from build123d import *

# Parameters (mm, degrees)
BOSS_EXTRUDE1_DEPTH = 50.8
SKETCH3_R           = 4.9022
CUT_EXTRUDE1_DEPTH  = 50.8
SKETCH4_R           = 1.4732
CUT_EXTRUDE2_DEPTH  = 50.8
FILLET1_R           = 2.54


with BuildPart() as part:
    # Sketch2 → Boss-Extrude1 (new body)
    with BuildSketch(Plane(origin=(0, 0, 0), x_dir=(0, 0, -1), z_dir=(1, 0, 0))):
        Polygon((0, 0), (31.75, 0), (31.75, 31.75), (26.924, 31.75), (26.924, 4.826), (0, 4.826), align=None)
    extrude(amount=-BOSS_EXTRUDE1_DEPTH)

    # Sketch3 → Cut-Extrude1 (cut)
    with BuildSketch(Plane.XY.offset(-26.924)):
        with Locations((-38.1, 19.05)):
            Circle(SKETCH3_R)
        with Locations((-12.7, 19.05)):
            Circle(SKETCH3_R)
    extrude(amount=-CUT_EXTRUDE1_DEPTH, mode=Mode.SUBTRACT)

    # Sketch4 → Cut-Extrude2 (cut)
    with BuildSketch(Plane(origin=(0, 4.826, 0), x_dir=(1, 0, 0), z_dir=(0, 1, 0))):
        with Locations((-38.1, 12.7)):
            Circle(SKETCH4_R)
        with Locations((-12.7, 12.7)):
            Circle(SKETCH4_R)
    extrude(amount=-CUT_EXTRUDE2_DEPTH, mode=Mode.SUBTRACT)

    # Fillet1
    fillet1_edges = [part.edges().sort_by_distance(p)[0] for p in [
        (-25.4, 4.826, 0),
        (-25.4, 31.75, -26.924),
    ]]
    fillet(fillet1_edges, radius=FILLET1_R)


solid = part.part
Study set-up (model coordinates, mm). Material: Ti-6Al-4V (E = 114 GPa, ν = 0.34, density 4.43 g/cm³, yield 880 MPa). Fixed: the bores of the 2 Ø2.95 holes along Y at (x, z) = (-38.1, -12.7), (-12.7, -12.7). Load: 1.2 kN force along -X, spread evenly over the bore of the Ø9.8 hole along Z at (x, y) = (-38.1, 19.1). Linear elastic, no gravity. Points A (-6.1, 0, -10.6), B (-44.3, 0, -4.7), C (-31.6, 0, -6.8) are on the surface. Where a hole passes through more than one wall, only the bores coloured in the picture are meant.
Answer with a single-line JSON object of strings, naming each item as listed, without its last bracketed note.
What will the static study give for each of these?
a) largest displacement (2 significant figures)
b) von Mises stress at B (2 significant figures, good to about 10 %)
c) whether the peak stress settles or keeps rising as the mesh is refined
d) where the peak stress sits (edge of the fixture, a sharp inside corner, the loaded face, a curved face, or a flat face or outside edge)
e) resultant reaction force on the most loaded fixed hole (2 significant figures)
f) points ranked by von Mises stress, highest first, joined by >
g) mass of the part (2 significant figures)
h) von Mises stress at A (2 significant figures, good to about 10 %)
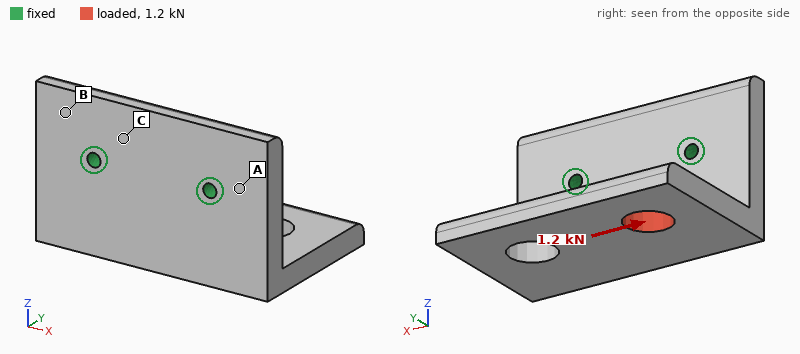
{"largest displacement": "72 µm", "von Mises stress at B": "21 MPa", "whether the peak stress settles or keeps rising as the mesh is refined": "keeps rising", "where the peak stress sits": "edge of the fixture", "resultant reaction force on the most loaded fixed hole": "1.1 kN", "points ranked by von Mises stress, highest first, joined by >": "A > B > C", "mass of the part": "60 g", "von Mises stress at A": "37 MPa"}
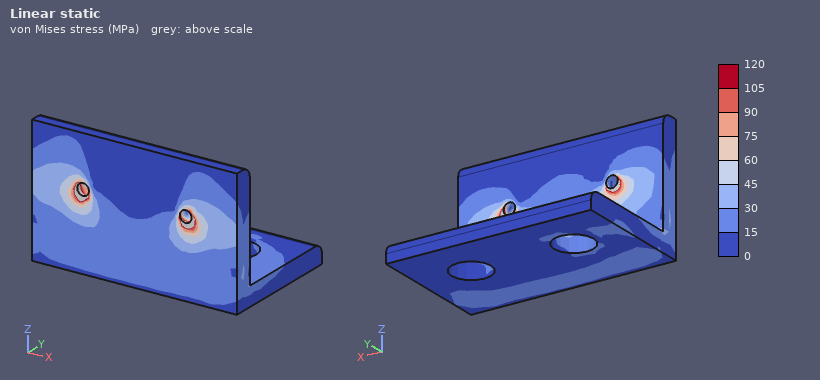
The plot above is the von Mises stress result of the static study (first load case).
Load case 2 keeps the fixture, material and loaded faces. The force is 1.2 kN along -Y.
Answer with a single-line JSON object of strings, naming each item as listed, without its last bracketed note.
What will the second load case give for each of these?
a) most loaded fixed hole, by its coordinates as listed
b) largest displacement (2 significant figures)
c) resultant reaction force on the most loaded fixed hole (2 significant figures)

{"most loaded fixed hole, by its coordinates as listed": "(-38.1, -12.7)", "largest displacement": "0.17 mm", "resultant reaction force on the most loaded fixed hole": "1.1 kN"}
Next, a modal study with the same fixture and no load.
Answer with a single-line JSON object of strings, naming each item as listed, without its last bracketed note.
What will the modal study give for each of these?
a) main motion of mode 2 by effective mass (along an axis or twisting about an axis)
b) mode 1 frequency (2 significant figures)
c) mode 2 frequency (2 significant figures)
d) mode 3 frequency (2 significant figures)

{"main motion of mode 2 by effective mass": "along X", "mode 1 frequency": "2400 Hz", "mode 2 frequency": "4100 Hz", "mode 3 frequency": "6800 Hz"}
